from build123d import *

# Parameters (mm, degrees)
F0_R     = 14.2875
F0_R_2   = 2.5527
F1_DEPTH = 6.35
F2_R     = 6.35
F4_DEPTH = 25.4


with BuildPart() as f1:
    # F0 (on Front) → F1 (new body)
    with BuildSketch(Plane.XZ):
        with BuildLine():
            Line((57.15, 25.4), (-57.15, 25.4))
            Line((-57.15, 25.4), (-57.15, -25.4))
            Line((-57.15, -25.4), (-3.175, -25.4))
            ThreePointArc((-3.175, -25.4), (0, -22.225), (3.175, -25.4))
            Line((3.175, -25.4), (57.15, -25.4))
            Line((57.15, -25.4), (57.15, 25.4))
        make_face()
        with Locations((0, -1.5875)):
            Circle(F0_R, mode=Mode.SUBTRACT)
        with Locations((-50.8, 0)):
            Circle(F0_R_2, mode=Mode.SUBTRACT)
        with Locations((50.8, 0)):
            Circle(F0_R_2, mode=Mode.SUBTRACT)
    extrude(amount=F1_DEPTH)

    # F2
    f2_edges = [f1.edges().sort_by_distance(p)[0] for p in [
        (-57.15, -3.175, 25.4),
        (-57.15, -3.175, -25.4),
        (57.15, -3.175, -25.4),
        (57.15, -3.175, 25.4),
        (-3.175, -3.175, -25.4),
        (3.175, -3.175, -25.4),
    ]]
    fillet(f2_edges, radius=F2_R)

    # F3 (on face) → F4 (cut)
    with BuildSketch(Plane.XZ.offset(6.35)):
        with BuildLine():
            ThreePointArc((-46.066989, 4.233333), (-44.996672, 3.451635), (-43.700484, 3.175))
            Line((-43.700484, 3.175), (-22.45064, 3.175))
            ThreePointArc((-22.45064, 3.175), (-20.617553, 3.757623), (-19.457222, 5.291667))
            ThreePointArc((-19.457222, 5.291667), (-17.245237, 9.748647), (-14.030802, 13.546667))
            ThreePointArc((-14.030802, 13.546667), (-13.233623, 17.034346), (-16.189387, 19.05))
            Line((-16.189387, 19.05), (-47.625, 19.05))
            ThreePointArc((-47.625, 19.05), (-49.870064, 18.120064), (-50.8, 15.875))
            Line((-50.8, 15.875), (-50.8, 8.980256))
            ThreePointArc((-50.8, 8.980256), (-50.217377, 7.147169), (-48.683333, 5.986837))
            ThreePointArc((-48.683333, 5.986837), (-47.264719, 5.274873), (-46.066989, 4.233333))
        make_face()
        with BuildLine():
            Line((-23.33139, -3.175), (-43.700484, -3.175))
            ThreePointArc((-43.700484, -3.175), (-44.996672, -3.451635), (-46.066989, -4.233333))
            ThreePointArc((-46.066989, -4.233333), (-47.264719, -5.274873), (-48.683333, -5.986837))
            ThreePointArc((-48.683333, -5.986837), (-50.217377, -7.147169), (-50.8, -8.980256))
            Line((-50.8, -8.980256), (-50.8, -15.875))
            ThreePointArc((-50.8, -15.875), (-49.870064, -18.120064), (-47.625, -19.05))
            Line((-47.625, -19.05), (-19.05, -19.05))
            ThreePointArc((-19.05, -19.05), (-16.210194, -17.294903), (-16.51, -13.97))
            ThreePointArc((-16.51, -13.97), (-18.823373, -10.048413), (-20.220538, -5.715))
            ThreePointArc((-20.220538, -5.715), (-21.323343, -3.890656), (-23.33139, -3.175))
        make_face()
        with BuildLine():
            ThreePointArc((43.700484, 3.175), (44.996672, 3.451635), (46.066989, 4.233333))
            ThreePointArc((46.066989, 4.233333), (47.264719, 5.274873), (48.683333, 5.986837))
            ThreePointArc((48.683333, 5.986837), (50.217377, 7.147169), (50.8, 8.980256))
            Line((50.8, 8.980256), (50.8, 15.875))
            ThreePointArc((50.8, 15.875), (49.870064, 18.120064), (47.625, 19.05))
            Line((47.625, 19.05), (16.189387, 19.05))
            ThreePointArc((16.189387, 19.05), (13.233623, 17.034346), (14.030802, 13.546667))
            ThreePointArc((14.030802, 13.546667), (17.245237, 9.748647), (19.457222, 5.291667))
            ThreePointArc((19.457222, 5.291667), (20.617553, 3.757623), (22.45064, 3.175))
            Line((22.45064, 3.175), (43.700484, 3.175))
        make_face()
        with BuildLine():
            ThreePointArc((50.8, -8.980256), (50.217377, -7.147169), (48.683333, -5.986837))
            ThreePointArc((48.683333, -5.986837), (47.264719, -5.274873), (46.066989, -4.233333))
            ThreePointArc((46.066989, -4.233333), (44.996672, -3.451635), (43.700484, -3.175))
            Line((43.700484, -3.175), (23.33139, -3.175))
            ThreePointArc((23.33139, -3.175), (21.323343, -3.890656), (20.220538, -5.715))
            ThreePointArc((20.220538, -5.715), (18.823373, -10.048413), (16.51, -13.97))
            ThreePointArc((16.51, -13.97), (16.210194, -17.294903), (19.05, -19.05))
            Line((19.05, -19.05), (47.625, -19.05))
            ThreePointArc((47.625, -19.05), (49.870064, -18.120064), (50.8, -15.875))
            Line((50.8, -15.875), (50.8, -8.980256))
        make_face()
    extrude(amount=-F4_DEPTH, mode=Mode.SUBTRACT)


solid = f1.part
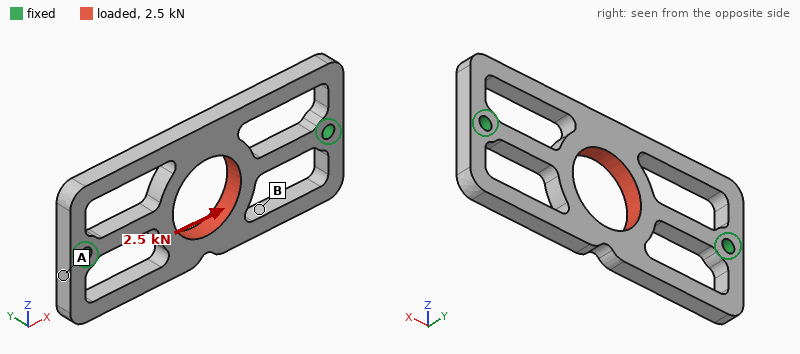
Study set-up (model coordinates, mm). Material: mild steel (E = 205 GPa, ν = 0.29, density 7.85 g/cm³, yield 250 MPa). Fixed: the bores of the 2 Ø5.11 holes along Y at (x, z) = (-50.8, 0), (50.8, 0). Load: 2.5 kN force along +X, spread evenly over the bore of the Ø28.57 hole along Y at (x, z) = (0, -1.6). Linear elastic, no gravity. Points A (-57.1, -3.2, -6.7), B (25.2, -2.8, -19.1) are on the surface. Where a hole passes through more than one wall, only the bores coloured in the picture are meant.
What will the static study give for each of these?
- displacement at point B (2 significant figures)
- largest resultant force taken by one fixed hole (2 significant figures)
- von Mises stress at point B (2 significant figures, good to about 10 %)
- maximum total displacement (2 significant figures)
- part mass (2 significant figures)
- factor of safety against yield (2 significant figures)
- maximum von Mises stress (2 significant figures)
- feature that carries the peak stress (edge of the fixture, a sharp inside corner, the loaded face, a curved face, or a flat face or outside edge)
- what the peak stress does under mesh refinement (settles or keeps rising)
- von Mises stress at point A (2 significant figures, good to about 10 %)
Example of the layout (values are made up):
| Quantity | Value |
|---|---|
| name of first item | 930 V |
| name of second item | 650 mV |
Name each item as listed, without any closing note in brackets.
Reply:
| Quantity | Value |
|---|---|
| displacement at point B | 7.0 µm |
| largest resultant force taken by one fixed hole | 1.3 kN |
| von Mises stress at point B | 6.6 MPa |
| maximum total displacement | 7.3 µm |
| part mass | 150 g |
| factor of safety against yield | 4.6 |
| maximum von Mises stress | 55 MPa |
| feature that carries the peak stress | a curved face |
| what the peak stress does under mesh refinement | settles |
| von Mises stress at point A | 23 MPa |
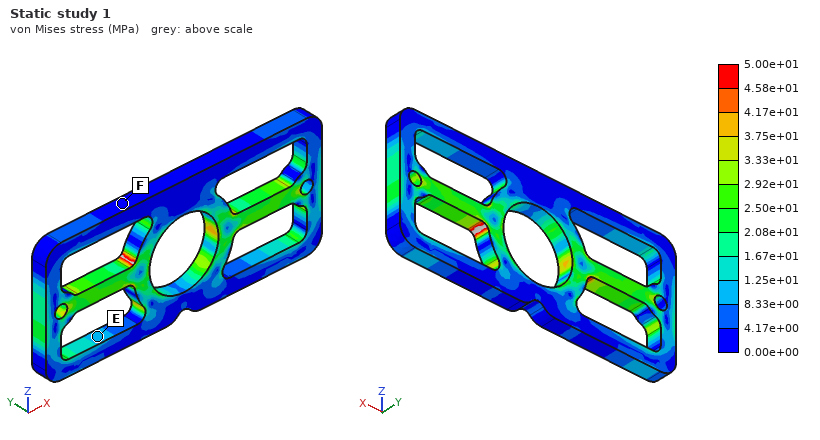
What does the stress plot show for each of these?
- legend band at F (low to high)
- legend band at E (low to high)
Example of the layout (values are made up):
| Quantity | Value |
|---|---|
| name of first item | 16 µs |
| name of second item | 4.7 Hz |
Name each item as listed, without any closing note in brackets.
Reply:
| Quantity | Value |
|---|---|
| legend band at F | 0.00e+00 to 4.17e+00 MPa |
| legend band at E | 8.33e+00 to 1.25e+01 MPa |
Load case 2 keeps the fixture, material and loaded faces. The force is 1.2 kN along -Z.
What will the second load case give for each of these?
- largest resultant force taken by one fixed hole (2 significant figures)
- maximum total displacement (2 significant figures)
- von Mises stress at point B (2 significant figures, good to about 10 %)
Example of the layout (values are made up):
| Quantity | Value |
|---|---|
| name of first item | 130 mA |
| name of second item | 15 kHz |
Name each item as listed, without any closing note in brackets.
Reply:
| Quantity | Value |
|---|---|
| largest resultant force taken by one fixed hole | 600 N |
| maximum total displacement | 32 µm |
| von Mises stress at point B | 21 MPa |
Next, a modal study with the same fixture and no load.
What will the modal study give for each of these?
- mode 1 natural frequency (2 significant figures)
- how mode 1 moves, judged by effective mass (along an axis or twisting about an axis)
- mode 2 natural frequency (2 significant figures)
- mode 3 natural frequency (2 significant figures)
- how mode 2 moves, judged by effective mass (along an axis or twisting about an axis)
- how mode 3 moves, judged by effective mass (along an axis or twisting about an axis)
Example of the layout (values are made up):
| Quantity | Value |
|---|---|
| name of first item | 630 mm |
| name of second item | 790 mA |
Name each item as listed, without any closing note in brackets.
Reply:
| Quantity | Value |
|---|---|
| mode 1 natural frequency | 2000 Hz |
| how mode 1 moves, judged by effective mass | along Y |
| mode 2 natural frequency | 2200 Hz |
| mode 3 natural frequency | 3600 Hz |
| how mode 2 moves, judged by effective mass | twisting about X |
| how mode 3 moves, judged by effective mass | along Z |
